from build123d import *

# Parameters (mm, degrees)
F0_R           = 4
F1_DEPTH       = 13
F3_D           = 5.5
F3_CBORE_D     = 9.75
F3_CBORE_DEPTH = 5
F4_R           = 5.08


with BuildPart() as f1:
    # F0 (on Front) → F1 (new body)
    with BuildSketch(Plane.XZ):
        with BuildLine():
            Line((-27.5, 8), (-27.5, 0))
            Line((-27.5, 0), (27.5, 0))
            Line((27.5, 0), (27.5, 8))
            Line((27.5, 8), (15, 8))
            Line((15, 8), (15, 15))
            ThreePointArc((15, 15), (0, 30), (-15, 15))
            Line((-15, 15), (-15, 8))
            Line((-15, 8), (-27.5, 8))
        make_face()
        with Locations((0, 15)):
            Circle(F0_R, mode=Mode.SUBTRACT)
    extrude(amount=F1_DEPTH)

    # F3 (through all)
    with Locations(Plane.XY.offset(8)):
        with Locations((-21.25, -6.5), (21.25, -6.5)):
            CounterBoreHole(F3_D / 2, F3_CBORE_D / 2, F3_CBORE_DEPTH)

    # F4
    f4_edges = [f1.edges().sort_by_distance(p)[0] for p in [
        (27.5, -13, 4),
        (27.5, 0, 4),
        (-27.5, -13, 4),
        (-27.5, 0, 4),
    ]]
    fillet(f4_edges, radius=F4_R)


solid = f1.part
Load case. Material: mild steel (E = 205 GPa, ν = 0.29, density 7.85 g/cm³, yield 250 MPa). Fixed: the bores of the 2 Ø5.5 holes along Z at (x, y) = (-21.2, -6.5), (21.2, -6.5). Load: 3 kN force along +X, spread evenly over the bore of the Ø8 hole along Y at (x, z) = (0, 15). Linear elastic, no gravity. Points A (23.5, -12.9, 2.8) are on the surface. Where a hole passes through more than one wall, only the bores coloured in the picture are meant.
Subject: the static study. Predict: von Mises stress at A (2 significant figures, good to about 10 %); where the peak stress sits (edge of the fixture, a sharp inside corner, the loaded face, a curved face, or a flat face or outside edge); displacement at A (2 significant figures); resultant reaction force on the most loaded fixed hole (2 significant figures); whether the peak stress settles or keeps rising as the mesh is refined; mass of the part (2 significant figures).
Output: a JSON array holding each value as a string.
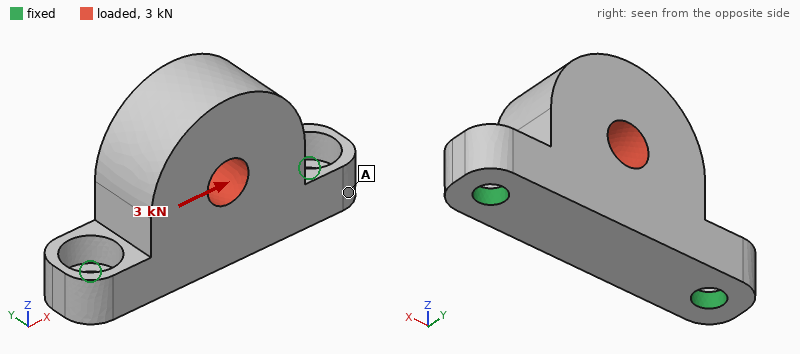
["14 MPa", "edge of the fixture", "1.1 µm", "1.8 kN", "keeps rising", "89 g"]
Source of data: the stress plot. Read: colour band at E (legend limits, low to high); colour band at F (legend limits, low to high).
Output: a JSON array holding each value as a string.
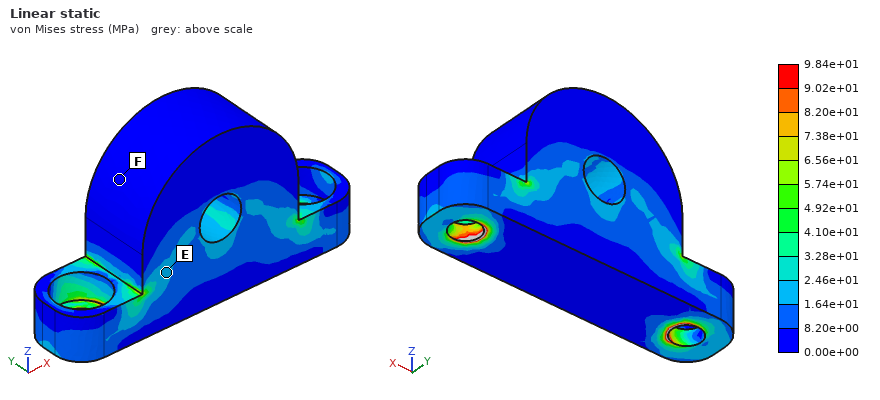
["1.64e+01 to 2.46e+01 MPa", "0.00e+00 to 8.20e+00 MPa"]
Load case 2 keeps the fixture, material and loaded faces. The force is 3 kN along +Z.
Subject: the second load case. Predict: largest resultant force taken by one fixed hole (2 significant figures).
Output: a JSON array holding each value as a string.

["1.8 kN"]
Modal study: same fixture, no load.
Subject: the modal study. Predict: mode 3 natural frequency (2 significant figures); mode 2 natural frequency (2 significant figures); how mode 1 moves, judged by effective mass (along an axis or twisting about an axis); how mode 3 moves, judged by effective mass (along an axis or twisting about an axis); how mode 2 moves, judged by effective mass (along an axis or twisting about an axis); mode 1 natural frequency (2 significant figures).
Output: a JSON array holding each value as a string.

["15 kHz", "14 kHz", "along Y", "along X", "along Z", "4000 Hz"]
